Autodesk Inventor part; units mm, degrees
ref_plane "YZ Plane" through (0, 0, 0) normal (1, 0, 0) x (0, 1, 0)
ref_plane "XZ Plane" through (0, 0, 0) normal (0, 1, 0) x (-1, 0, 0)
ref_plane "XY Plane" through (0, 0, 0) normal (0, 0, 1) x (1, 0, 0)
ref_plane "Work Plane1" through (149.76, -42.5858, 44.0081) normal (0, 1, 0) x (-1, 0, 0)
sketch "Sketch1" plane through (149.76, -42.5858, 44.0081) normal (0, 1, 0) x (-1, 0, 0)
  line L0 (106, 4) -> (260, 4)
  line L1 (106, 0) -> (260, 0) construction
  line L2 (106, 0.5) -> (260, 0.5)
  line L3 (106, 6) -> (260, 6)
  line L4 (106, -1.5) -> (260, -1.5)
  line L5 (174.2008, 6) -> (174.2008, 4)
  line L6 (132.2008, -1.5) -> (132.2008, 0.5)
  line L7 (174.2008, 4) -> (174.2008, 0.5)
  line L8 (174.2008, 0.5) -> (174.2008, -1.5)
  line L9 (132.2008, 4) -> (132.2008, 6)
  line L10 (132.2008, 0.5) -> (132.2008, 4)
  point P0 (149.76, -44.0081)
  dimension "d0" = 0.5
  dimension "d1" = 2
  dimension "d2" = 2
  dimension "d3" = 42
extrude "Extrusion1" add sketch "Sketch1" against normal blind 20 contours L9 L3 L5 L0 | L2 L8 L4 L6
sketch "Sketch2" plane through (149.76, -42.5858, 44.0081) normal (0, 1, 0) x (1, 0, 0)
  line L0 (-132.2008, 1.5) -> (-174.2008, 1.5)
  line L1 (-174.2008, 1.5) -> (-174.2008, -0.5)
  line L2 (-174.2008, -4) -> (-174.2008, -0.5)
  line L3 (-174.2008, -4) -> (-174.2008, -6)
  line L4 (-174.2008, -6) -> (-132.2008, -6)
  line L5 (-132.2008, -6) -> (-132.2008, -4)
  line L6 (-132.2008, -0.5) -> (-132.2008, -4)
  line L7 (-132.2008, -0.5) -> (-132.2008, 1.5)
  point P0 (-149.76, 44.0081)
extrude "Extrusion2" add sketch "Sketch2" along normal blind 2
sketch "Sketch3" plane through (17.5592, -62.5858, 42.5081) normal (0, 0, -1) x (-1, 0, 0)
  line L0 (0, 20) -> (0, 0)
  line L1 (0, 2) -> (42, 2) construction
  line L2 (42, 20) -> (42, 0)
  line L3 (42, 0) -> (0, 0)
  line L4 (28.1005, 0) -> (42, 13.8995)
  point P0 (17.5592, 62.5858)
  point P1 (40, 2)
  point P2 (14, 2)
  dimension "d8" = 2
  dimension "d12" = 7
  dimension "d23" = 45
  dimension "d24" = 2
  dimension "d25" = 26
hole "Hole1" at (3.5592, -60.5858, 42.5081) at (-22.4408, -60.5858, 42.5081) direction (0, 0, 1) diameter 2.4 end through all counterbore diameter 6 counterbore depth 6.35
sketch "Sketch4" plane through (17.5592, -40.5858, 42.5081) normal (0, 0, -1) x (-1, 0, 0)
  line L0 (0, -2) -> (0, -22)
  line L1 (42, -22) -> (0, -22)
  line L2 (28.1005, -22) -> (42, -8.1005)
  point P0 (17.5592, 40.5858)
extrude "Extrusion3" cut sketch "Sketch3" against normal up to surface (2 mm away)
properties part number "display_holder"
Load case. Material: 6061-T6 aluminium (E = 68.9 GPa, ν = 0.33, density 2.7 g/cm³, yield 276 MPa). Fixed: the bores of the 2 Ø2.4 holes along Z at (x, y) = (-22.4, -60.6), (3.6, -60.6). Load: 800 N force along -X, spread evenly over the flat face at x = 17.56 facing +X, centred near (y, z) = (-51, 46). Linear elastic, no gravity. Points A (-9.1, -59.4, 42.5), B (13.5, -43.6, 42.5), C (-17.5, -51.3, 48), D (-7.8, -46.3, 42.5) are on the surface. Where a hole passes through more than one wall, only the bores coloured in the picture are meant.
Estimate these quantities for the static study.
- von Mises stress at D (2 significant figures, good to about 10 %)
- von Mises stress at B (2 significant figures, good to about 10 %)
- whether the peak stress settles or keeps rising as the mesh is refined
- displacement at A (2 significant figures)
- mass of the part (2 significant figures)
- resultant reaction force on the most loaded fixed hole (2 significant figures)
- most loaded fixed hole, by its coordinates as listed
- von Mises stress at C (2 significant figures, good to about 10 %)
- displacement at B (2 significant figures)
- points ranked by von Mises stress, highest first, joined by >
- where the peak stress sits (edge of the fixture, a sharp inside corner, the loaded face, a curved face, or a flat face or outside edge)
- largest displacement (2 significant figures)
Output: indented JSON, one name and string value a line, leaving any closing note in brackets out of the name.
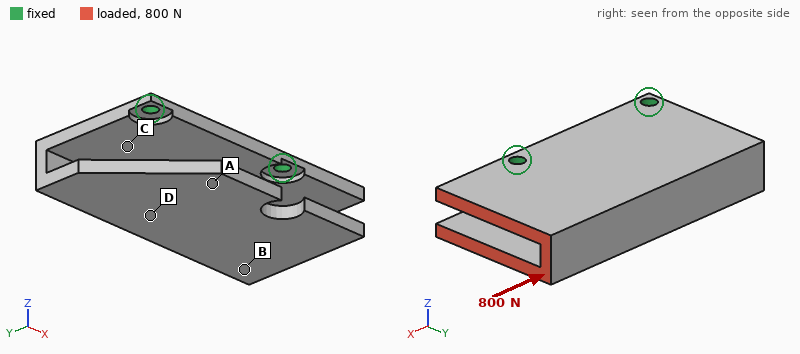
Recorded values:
{
  "von Mises stress at D": "26 MPa",
  "von Mises stress at B": "46 MPa",
  "whether the peak stress settles or keeps rising as the mesh is refined": "keeps rising",
  "displacement at A": "0.13 mm",
  "mass of the part": "10.0 g",
  "resultant reaction force on the most loaded fixed hole": "560 N",
  "most loaded fixed hole, by its coordinates as listed": "(3.6, -60.6)",
  "von Mises stress at C": "81 MPa",
  "displacement at B": "0.22 mm",
  "points ranked by von Mises stress, highest first, joined by >": "C > B > D > A",
  "where the peak stress sits": "edge of the fixture",
  "largest displacement": "0.28 mm"
}
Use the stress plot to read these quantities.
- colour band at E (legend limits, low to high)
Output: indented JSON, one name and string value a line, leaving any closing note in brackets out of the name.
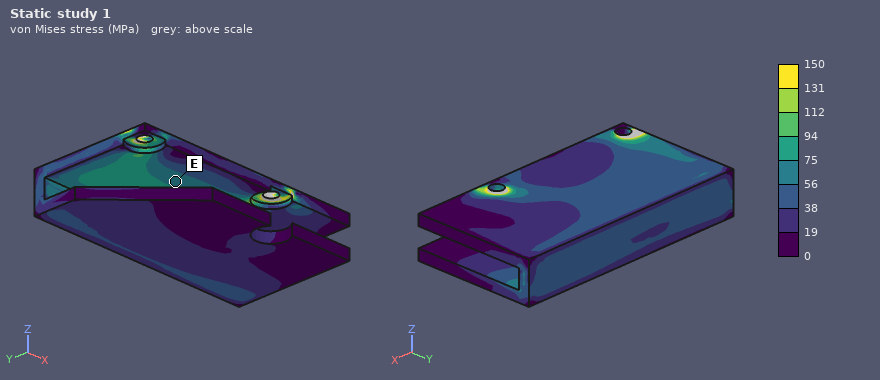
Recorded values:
{
  "colour band at E": "56 to 75 MPa"
}
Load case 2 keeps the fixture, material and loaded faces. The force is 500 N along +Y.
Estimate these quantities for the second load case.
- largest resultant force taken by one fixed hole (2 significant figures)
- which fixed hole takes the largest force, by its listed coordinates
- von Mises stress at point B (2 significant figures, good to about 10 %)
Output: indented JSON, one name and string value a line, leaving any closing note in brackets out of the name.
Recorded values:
{
  "largest resultant force taken by one fixed hole": "760 N",
  "which fixed hole takes the largest force, by its listed coordinates": "(3.6, -60.6)",
  "von Mises stress at point B": "40 MPa"
}
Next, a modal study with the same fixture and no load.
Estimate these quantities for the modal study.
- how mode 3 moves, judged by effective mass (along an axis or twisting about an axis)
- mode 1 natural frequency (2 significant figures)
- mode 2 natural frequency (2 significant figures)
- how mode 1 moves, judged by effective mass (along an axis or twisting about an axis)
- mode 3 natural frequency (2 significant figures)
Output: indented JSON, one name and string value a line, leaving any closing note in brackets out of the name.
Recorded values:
{
  "how mode 3 moves, judged by effective mass": "along Z",
  "mode 1 natural frequency": "1300 Hz",
  "mode 2 natural frequency": "2200 Hz",
  "how mode 1 moves, judged by effective mass": "along Z",
  "mode 3 natural frequency": "2700 Hz"
}
